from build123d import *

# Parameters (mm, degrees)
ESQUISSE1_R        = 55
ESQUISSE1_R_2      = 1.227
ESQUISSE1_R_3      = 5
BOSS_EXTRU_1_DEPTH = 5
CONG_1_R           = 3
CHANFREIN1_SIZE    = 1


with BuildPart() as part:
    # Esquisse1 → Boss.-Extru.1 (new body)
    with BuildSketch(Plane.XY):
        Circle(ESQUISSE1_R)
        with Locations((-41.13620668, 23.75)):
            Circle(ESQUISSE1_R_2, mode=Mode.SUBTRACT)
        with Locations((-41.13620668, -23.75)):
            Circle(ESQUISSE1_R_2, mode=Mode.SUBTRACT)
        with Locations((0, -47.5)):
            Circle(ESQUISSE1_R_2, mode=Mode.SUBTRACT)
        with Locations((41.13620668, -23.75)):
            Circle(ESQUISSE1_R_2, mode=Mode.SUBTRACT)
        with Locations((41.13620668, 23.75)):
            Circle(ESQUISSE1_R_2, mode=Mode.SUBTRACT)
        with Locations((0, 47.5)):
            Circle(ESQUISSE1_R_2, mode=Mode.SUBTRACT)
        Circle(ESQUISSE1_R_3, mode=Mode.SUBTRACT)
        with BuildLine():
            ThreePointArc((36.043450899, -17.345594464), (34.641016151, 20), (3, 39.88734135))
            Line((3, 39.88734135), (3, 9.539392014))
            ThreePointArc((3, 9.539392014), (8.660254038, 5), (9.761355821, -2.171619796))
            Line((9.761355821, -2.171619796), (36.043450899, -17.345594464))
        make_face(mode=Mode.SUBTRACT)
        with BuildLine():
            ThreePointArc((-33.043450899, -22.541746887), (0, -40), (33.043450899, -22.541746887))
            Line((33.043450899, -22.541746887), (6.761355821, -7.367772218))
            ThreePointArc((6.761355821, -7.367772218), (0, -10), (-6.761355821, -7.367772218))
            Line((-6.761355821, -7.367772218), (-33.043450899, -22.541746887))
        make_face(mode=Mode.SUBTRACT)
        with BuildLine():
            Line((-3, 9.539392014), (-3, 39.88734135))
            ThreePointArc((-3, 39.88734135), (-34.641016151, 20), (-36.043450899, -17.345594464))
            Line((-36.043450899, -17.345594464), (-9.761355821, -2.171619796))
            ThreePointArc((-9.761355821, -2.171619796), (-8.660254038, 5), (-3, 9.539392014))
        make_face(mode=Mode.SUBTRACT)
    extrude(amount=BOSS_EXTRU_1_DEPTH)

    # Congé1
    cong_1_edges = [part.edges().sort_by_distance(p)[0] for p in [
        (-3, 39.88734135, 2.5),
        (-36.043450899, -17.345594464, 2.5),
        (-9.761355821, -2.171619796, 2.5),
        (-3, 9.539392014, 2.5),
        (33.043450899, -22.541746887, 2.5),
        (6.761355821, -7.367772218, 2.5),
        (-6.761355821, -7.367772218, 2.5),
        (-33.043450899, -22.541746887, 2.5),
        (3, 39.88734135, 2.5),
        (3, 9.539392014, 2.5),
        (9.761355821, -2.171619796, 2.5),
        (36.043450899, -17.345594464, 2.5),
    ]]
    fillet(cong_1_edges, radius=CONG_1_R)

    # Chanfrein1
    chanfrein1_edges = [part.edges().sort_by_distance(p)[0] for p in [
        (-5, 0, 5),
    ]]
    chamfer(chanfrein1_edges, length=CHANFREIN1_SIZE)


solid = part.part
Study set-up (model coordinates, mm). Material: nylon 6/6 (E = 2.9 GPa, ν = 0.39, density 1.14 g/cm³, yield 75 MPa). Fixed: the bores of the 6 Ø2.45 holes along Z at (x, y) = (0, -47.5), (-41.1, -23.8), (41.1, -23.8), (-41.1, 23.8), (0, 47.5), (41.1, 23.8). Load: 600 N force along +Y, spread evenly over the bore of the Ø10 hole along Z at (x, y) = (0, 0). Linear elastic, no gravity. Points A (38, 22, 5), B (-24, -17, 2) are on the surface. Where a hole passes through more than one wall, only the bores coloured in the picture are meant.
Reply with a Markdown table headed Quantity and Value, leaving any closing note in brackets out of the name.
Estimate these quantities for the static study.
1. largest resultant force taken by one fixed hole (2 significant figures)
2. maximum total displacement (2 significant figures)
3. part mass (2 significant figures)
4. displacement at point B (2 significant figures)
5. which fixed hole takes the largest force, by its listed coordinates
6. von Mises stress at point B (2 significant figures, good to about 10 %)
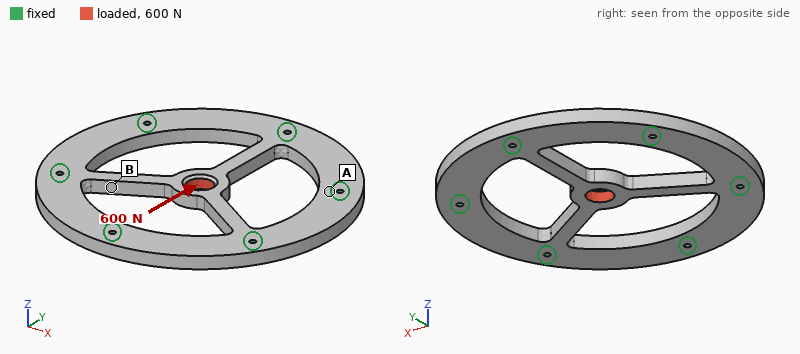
| Quantity | Value |
|---|---|
| largest resultant force taken by one fixed hole | 360 N |
| maximum total displacement | 0.32 mm |
| part mass | 30 g |
| displacement at point B | 0.070 mm |
| which fixed hole takes the largest force, by its listed coordinates | (0, 47.5) |
| von Mises stress at point B | 10 MPa |
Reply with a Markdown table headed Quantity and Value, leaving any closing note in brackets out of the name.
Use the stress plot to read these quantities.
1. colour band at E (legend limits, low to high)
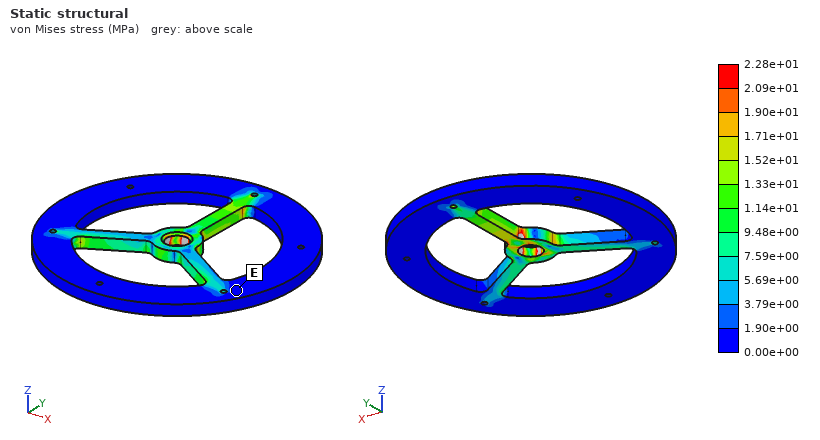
| Quantity | Value |
|---|---|
| colour band at E | 0.00e+00 to 1.90e+00 MPa |
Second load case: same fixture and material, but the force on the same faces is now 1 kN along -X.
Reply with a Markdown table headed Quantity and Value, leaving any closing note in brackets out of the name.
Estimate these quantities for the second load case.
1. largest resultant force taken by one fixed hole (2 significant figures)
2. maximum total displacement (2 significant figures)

| Quantity | Value |
|---|---|
| largest resultant force taken by one fixed hole | 520 N |
| maximum total displacement | 0.50 mm |
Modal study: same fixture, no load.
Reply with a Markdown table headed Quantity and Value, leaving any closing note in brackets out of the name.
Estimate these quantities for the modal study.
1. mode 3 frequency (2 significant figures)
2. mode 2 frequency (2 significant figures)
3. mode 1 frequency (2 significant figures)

| Quantity | Value |
|---|---|
| mode 3 frequency | 2600 Hz |
| mode 2 frequency | 2500 Hz |
| mode 1 frequency | 1000 Hz |
